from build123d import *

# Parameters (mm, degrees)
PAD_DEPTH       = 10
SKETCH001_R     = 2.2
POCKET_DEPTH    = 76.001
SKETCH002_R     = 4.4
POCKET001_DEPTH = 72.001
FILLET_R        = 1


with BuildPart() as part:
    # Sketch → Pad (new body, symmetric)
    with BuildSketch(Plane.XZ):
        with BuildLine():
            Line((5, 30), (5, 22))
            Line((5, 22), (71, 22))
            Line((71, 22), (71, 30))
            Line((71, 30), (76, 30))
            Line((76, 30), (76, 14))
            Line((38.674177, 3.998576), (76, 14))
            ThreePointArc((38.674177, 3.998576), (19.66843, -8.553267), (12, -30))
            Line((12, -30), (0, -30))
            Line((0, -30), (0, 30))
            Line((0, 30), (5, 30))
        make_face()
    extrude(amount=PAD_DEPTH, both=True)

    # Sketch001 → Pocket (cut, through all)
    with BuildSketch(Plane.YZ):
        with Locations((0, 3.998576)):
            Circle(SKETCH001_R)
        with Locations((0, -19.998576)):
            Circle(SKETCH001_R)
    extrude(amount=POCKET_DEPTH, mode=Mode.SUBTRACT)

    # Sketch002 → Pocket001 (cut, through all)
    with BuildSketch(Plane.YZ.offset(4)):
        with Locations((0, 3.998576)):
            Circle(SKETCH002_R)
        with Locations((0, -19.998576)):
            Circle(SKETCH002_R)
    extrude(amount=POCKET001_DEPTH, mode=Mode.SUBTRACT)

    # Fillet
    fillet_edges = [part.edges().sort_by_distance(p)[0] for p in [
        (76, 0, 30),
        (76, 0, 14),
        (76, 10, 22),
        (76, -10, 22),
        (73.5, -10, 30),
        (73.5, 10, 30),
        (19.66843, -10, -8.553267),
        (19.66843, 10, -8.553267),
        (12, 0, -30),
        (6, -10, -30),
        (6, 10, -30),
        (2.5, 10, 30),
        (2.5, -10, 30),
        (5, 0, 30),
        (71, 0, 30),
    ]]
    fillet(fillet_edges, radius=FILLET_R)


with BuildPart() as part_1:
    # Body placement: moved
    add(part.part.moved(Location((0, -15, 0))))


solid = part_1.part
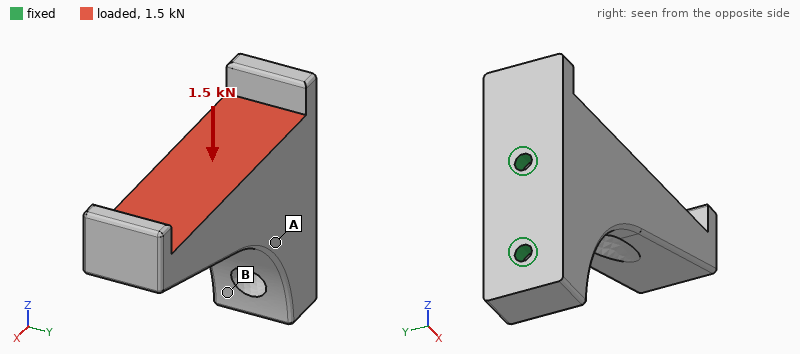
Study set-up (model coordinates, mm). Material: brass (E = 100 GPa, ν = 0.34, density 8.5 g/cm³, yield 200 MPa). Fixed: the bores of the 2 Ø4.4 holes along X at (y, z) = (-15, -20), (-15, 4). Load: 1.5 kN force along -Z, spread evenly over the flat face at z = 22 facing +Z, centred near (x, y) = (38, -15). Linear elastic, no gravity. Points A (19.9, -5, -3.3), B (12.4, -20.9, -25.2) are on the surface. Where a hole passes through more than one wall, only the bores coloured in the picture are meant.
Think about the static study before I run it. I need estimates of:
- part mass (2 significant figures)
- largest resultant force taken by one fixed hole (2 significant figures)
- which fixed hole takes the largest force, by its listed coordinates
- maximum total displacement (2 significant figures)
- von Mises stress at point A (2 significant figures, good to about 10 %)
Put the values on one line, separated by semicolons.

300 g; 2.5 kN; (-15, -20); 73 µm; 19 MPa
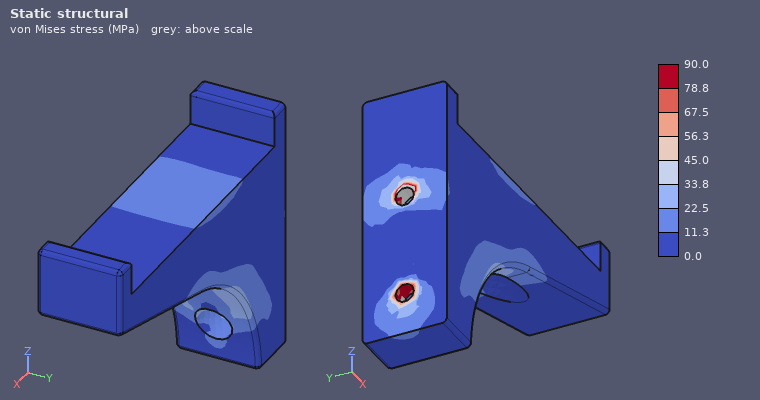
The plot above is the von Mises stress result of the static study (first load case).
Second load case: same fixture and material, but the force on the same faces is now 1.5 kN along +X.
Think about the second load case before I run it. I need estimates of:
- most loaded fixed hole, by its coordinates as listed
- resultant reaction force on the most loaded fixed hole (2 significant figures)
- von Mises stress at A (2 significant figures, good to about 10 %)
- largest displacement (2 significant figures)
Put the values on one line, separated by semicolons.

(-15, 4); 2.5 kN; 8.8 MPa; 49 µm
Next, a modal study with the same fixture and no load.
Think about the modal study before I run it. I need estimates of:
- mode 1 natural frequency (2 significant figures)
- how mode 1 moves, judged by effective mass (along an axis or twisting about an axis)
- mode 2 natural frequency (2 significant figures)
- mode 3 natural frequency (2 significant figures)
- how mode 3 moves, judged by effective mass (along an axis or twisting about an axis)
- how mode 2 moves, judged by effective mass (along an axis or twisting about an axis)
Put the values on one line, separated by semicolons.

930 Hz; along Y; 2000 Hz; 6200 Hz; along X; along Z
